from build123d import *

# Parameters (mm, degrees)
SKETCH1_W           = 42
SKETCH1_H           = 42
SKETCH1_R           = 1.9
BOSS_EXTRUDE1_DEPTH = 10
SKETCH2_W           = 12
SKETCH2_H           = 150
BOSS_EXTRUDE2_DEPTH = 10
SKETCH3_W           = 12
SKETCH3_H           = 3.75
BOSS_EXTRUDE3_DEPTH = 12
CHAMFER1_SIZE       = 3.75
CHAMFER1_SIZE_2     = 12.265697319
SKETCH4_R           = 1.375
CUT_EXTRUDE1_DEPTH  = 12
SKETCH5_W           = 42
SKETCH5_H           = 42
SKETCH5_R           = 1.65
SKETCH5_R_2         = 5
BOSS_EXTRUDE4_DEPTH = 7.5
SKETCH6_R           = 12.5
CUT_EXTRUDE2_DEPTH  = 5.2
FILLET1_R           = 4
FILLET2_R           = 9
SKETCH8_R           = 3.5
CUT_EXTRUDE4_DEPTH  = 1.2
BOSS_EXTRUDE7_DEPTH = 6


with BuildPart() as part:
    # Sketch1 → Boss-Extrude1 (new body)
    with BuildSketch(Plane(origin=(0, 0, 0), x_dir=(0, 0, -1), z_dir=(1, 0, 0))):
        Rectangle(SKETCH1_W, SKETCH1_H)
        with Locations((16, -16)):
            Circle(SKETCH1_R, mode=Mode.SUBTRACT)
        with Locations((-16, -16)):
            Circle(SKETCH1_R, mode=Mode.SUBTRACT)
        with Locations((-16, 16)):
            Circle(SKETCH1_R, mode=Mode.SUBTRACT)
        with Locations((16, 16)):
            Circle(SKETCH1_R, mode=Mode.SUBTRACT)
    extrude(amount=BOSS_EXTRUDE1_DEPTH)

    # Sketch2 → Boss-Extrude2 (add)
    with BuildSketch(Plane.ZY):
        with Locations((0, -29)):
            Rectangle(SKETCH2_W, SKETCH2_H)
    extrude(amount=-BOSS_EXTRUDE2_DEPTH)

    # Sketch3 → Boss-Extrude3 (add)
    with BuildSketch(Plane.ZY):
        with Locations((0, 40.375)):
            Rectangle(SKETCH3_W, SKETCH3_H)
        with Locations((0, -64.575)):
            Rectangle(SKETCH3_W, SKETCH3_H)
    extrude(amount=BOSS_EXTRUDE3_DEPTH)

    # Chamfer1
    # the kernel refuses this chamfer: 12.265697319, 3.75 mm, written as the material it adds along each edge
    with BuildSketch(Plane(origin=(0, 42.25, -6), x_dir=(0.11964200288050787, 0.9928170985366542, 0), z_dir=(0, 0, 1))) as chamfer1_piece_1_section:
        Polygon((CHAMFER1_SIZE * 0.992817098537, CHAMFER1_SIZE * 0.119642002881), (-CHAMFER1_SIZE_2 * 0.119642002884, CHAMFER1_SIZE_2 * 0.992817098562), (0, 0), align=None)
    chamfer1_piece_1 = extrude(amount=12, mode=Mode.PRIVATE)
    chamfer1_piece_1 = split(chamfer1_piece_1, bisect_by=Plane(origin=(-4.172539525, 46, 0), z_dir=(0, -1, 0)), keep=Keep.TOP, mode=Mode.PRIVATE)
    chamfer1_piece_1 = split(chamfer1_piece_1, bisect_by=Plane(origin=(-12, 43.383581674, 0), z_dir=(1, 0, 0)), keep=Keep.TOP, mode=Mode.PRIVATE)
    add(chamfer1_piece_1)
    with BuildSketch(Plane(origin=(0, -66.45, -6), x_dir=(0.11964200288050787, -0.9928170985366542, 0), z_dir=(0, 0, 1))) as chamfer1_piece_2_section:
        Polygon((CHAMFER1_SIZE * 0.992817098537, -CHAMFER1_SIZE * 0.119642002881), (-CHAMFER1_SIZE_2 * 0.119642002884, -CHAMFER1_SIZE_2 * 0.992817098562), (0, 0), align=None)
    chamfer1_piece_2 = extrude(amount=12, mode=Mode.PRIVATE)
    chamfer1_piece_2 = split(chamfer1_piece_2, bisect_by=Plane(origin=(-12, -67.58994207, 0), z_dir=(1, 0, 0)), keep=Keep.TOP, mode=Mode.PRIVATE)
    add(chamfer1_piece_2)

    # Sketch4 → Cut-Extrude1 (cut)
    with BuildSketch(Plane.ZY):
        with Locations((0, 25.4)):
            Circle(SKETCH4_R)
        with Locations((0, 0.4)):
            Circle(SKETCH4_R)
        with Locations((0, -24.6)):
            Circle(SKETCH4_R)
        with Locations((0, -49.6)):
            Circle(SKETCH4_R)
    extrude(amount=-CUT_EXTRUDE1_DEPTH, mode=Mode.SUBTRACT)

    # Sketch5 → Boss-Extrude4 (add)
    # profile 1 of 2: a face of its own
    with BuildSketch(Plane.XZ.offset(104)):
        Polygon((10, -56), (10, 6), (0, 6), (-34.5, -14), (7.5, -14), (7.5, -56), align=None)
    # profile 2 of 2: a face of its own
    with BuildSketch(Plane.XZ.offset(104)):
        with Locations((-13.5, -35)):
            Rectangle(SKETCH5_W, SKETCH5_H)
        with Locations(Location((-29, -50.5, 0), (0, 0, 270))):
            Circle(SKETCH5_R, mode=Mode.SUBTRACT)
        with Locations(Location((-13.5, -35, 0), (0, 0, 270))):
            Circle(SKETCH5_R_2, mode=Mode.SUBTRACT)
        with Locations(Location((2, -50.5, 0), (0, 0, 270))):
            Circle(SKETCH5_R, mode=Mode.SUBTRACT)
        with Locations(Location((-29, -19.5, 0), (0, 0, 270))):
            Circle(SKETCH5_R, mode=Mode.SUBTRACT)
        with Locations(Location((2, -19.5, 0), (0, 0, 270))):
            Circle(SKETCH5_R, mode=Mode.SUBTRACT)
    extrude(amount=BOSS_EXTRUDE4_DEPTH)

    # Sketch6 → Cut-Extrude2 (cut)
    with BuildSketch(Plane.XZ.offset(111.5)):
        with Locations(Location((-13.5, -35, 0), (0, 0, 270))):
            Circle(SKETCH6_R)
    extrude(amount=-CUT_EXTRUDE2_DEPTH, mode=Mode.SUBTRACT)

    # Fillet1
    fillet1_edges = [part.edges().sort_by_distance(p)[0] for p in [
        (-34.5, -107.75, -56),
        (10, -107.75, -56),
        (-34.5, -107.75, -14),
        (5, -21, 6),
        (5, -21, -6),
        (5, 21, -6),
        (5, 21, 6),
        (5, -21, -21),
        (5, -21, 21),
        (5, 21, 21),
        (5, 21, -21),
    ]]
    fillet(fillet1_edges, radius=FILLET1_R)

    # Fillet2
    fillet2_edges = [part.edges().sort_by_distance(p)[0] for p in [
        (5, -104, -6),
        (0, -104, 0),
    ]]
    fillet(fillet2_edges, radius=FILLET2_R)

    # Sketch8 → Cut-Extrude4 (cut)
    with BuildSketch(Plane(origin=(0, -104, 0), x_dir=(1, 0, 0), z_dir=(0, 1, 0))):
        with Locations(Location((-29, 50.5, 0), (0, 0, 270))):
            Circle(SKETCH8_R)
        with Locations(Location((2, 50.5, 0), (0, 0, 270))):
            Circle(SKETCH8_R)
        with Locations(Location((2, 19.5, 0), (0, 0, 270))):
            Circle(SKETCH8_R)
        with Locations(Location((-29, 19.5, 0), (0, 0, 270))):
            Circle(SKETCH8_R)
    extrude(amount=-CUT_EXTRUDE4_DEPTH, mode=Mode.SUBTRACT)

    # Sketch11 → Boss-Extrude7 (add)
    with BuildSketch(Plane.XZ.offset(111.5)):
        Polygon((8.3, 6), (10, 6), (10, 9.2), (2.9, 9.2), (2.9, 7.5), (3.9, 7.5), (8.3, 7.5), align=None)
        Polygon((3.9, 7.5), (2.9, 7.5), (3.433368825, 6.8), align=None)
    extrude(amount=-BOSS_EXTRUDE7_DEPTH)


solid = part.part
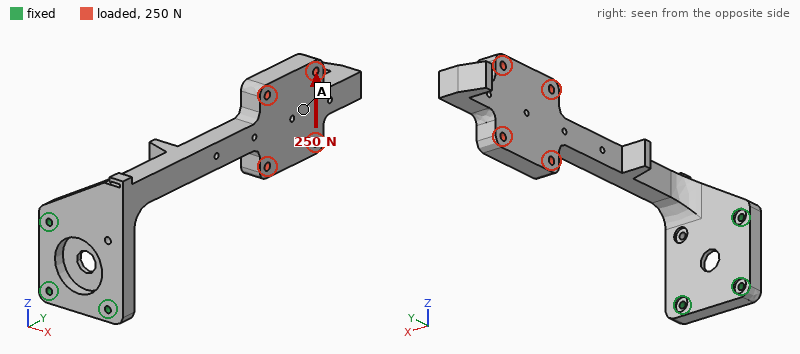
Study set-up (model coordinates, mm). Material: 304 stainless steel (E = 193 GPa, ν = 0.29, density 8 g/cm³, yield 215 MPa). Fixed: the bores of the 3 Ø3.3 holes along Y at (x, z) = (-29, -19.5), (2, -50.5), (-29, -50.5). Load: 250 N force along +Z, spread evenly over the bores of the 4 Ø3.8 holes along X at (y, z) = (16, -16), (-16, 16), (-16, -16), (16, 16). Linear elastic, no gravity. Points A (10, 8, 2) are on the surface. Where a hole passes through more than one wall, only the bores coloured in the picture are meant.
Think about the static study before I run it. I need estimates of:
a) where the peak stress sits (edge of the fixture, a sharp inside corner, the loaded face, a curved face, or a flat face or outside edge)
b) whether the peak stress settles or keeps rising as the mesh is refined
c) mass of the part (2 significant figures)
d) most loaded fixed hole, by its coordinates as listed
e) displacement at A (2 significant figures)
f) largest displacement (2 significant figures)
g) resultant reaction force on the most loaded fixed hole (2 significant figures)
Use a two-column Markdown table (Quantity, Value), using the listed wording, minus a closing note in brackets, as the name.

| Quantity | Value |
|---|---|
| where the peak stress sits | edge of the fixture |
| whether the peak stress settles or keeps rising as the mesh is refined | keeps rising |
| mass of the part | 380 g |
| most loaded fixed hole, by its coordinates as listed | (-29, -19.5) |
| displacement at A | 0.80 mm |
| largest displacement | 1.1 mm |
| resultant reaction force on the most loaded fixed hole | 660 N |
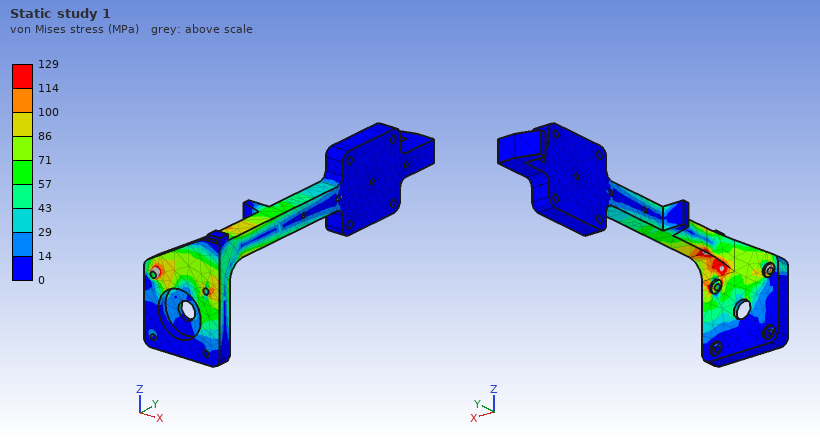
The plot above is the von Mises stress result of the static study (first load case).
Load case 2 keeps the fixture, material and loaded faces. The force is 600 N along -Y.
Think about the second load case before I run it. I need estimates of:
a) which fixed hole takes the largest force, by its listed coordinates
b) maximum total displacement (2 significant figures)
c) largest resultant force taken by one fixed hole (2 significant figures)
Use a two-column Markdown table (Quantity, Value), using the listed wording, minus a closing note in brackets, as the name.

| Quantity | Value |
|---|---|
| which fixed hole takes the largest force, by its listed coordinates | (-29, -19.5) |
| maximum total displacement | 0.38 mm |
| largest resultant force taken by one fixed hole | 690 N |
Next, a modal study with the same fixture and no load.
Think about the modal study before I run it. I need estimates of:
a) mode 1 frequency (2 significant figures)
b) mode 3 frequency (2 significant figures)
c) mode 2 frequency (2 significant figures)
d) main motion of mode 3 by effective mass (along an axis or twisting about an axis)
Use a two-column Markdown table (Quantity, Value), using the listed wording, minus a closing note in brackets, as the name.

| Quantity | Value |
|---|---|
| mode 1 frequency | 180 Hz |
| mode 3 frequency | 1100 Hz |
| mode 2 frequency | 220 Hz |
| main motion of mode 3 by effective mass | along Y |
